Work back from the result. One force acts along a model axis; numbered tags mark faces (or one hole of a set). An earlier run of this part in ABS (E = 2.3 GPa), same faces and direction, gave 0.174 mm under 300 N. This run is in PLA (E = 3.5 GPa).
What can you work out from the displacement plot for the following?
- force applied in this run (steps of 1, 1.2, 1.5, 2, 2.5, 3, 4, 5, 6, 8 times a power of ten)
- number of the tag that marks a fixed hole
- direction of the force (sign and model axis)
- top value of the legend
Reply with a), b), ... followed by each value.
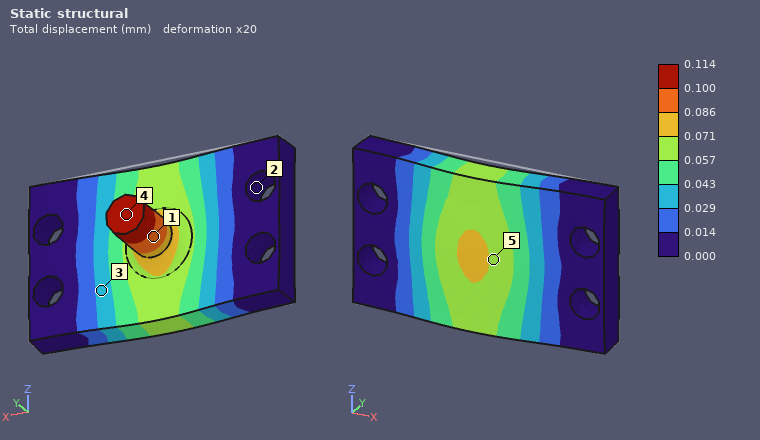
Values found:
a) 300 N
b) 2
c) -Y
d) 0.114 mm
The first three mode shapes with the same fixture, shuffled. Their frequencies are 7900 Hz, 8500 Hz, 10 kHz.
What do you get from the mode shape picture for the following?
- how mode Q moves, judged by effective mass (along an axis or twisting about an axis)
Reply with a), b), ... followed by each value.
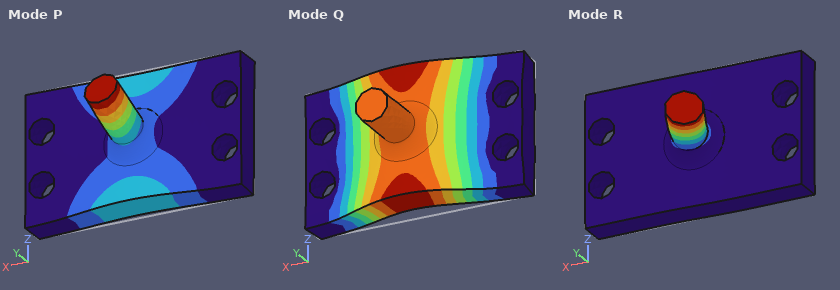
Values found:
a) along Y
